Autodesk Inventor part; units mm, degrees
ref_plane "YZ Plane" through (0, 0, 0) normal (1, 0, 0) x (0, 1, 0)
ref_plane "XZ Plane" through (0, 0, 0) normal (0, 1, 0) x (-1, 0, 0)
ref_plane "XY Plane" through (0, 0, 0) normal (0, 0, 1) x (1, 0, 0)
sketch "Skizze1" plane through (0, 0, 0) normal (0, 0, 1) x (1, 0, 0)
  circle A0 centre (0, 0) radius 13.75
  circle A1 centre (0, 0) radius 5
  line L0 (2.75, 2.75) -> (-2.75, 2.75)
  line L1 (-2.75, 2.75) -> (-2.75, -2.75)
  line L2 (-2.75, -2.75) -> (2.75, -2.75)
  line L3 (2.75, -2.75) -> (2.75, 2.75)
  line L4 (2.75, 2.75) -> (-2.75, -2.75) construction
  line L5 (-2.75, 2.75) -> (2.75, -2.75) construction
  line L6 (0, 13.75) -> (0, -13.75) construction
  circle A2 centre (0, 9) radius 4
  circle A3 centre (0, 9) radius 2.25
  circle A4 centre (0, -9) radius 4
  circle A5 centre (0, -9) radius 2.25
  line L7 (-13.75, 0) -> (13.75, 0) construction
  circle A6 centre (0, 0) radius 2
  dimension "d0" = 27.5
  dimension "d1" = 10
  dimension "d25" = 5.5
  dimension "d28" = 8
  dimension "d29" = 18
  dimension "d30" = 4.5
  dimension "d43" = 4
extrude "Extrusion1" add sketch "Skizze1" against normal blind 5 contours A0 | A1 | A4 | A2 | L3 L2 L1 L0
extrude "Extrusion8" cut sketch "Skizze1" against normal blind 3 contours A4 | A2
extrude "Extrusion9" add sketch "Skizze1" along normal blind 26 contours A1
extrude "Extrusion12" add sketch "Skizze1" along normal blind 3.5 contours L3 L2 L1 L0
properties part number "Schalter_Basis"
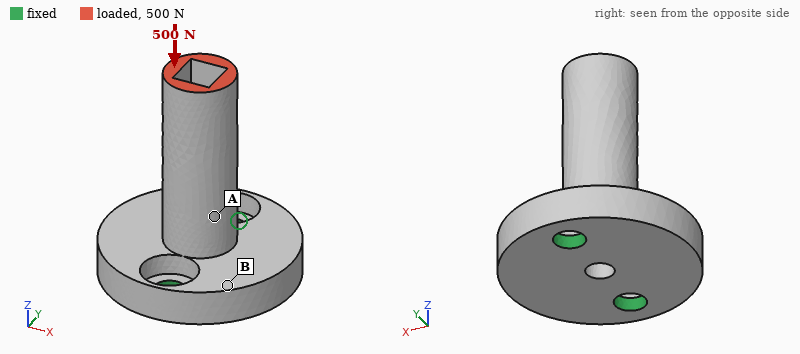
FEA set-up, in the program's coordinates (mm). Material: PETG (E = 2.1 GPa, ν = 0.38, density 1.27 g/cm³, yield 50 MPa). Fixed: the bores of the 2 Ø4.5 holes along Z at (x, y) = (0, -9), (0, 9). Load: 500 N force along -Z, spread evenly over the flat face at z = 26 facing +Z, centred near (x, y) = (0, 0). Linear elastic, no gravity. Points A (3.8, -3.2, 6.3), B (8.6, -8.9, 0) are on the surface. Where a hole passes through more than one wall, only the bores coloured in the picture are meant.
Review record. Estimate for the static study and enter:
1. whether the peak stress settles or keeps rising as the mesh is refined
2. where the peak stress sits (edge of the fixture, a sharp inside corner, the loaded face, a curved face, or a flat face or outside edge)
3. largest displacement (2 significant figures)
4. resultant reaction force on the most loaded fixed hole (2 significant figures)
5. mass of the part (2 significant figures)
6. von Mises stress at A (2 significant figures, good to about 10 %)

keeps rising
edge of the fixture
0.22 mm
270 N
4.9 g
10 MPa
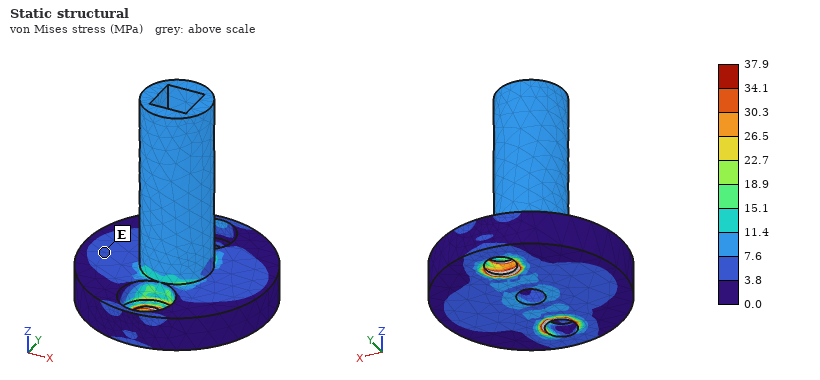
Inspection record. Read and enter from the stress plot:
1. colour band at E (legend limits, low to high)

3.8 to 7.6 MPa
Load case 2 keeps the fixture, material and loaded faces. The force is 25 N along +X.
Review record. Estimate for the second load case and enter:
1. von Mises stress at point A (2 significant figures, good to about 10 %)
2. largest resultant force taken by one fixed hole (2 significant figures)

4.6 MPa
13 N
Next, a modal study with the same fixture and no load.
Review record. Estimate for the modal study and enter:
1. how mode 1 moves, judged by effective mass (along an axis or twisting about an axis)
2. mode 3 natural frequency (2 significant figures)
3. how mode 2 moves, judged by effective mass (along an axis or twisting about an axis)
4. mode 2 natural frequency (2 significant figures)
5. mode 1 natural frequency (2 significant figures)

along X
4800 Hz
along Y
2100 Hz
1300 Hz
